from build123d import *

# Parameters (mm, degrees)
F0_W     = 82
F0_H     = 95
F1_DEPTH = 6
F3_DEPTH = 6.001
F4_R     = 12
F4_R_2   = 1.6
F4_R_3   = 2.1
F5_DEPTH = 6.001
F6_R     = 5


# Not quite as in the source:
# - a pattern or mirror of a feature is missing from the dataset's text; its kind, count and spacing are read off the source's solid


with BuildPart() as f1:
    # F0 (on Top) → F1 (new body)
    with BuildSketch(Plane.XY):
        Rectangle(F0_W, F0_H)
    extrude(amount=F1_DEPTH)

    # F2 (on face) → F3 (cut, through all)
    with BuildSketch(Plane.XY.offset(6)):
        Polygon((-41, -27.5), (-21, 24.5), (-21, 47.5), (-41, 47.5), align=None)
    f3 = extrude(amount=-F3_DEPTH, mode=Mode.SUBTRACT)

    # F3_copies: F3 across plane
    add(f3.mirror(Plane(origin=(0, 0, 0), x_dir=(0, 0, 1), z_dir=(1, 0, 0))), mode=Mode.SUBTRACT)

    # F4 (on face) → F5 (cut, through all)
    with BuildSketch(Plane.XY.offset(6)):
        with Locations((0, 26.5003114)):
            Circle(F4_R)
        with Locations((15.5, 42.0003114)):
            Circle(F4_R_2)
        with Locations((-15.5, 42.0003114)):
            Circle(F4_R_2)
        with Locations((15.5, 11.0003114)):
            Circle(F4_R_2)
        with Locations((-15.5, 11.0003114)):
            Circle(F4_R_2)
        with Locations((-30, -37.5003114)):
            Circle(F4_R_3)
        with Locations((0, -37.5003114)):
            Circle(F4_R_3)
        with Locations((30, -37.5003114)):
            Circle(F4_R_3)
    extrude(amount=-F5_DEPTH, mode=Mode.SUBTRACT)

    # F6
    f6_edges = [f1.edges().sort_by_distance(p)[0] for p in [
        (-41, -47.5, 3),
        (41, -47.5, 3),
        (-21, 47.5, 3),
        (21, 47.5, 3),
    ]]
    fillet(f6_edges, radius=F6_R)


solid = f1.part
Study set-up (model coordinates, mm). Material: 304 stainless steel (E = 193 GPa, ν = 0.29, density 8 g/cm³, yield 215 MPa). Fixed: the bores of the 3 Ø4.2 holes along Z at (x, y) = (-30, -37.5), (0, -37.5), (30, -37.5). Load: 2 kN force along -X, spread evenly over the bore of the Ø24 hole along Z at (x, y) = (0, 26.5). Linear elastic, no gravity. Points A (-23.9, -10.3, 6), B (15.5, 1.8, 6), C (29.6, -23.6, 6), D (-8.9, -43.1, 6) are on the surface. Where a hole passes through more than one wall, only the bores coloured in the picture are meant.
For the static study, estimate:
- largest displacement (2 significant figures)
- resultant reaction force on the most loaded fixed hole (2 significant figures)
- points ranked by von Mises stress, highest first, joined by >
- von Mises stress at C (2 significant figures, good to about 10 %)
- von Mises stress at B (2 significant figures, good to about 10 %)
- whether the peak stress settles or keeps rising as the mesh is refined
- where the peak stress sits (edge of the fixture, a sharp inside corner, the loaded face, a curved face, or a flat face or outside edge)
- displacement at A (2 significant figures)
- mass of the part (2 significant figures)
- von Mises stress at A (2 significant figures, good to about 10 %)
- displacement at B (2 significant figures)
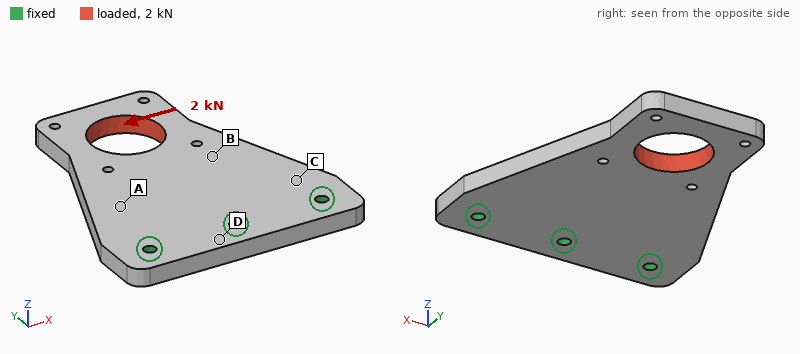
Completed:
20 µm
2.2 kN
C > A > B > D
17 MPa
7.8 MPa
keeps rising
edge of the fixture
3.5 µm
250 g
13 MPa
5.1 µm
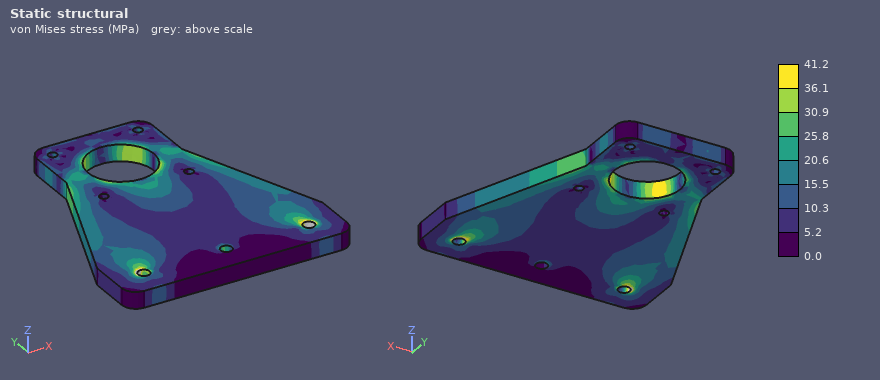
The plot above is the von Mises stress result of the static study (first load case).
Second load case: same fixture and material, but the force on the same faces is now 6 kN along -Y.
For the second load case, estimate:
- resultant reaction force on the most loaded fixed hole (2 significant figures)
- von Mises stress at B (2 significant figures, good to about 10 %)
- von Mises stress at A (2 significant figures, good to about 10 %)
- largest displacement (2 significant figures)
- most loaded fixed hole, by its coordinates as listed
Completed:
2.3 kN
17 MPa
15 MPa
12 µm
(0, -37.5)
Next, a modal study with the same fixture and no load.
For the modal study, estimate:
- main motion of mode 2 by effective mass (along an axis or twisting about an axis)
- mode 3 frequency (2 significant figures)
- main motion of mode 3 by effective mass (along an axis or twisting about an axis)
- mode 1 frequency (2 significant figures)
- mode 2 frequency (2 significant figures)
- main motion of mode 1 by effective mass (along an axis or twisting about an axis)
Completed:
twisting about Y
3700 Hz
along Z
920 Hz
3000 Hz
along Z
